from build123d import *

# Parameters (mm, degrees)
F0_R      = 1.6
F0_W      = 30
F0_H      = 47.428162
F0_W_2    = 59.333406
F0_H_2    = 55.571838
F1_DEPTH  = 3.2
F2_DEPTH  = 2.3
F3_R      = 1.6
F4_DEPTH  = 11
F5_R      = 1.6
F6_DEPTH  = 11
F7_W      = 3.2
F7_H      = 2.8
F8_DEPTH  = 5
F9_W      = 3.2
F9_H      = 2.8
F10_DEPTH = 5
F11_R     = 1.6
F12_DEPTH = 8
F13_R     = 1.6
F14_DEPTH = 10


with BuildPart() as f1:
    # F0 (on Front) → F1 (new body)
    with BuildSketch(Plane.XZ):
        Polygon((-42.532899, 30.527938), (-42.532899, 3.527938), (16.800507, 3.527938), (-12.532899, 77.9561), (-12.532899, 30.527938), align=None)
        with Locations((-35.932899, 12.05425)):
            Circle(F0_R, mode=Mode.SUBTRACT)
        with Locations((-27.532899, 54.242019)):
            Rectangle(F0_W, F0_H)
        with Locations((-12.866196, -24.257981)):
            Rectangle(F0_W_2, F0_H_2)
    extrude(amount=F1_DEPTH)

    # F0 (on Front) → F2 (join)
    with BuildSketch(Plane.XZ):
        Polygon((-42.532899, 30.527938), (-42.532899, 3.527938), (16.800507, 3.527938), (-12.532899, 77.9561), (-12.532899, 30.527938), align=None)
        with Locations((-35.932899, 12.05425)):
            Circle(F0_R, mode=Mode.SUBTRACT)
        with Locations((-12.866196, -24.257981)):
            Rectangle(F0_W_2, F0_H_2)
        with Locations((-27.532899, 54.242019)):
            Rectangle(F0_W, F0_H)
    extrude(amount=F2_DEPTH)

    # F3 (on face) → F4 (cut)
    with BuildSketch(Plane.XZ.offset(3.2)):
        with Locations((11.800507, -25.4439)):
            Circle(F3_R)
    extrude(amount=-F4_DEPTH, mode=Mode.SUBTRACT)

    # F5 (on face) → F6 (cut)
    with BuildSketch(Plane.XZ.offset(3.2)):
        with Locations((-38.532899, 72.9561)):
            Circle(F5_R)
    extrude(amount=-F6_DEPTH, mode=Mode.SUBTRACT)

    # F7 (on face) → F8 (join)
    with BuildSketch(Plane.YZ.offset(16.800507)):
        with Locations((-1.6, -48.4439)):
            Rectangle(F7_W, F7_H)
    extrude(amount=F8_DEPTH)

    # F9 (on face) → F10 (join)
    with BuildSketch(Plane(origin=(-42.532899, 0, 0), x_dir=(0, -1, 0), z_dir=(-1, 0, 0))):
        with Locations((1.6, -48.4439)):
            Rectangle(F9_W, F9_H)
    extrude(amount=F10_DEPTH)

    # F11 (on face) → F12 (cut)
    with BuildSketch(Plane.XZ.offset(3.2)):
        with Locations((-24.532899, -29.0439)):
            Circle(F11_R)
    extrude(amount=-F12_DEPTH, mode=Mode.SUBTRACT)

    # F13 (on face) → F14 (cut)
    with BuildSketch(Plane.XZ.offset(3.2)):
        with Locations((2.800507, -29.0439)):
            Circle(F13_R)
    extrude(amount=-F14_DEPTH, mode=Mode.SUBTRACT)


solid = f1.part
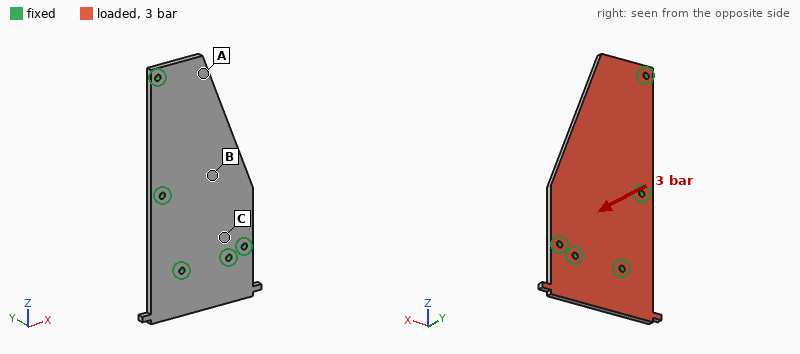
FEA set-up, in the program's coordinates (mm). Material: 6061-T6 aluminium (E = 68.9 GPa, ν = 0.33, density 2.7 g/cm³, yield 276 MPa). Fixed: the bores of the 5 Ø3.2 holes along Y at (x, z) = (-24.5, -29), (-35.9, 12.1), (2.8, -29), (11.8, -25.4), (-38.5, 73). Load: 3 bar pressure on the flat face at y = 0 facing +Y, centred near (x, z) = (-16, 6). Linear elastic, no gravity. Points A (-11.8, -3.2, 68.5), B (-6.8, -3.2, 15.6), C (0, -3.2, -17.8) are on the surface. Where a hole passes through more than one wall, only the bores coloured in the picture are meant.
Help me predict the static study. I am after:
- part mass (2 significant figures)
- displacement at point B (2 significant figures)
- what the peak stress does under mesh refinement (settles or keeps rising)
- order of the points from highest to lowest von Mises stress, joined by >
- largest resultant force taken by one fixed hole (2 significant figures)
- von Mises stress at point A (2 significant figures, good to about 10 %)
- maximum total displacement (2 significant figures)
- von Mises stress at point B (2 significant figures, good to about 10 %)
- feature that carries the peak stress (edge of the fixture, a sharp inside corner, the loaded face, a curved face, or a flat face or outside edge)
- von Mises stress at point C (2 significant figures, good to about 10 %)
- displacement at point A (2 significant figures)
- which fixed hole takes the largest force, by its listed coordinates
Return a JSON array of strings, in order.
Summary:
["57 g", "0.30 mm", "keeps rising", "C > B > A", "640 N", "18 MPa", "0.61 mm", "37 MPa", "edge of the fixture", "56 MPa", "0.35 mm", "(-35.9, 12.1)"]
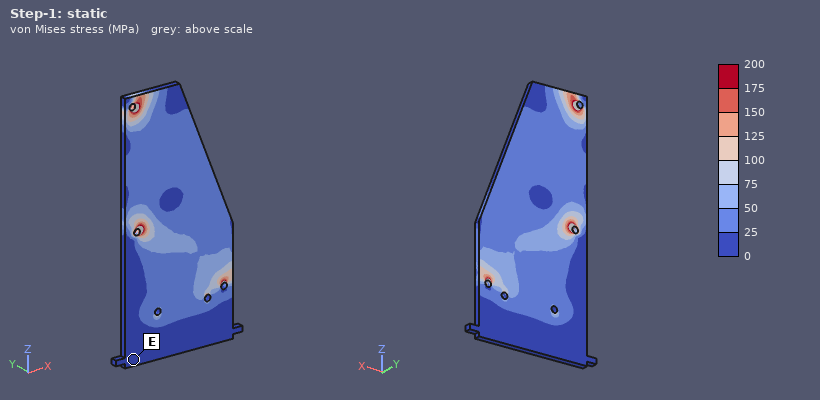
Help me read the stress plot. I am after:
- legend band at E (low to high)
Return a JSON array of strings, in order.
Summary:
["0 to 25 MPa"]
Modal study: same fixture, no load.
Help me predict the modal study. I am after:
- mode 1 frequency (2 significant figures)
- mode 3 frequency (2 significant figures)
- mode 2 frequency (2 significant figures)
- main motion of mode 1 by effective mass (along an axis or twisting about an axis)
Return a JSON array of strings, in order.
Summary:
["1600 Hz", "4200 Hz", "3400 Hz", "along Y"]
